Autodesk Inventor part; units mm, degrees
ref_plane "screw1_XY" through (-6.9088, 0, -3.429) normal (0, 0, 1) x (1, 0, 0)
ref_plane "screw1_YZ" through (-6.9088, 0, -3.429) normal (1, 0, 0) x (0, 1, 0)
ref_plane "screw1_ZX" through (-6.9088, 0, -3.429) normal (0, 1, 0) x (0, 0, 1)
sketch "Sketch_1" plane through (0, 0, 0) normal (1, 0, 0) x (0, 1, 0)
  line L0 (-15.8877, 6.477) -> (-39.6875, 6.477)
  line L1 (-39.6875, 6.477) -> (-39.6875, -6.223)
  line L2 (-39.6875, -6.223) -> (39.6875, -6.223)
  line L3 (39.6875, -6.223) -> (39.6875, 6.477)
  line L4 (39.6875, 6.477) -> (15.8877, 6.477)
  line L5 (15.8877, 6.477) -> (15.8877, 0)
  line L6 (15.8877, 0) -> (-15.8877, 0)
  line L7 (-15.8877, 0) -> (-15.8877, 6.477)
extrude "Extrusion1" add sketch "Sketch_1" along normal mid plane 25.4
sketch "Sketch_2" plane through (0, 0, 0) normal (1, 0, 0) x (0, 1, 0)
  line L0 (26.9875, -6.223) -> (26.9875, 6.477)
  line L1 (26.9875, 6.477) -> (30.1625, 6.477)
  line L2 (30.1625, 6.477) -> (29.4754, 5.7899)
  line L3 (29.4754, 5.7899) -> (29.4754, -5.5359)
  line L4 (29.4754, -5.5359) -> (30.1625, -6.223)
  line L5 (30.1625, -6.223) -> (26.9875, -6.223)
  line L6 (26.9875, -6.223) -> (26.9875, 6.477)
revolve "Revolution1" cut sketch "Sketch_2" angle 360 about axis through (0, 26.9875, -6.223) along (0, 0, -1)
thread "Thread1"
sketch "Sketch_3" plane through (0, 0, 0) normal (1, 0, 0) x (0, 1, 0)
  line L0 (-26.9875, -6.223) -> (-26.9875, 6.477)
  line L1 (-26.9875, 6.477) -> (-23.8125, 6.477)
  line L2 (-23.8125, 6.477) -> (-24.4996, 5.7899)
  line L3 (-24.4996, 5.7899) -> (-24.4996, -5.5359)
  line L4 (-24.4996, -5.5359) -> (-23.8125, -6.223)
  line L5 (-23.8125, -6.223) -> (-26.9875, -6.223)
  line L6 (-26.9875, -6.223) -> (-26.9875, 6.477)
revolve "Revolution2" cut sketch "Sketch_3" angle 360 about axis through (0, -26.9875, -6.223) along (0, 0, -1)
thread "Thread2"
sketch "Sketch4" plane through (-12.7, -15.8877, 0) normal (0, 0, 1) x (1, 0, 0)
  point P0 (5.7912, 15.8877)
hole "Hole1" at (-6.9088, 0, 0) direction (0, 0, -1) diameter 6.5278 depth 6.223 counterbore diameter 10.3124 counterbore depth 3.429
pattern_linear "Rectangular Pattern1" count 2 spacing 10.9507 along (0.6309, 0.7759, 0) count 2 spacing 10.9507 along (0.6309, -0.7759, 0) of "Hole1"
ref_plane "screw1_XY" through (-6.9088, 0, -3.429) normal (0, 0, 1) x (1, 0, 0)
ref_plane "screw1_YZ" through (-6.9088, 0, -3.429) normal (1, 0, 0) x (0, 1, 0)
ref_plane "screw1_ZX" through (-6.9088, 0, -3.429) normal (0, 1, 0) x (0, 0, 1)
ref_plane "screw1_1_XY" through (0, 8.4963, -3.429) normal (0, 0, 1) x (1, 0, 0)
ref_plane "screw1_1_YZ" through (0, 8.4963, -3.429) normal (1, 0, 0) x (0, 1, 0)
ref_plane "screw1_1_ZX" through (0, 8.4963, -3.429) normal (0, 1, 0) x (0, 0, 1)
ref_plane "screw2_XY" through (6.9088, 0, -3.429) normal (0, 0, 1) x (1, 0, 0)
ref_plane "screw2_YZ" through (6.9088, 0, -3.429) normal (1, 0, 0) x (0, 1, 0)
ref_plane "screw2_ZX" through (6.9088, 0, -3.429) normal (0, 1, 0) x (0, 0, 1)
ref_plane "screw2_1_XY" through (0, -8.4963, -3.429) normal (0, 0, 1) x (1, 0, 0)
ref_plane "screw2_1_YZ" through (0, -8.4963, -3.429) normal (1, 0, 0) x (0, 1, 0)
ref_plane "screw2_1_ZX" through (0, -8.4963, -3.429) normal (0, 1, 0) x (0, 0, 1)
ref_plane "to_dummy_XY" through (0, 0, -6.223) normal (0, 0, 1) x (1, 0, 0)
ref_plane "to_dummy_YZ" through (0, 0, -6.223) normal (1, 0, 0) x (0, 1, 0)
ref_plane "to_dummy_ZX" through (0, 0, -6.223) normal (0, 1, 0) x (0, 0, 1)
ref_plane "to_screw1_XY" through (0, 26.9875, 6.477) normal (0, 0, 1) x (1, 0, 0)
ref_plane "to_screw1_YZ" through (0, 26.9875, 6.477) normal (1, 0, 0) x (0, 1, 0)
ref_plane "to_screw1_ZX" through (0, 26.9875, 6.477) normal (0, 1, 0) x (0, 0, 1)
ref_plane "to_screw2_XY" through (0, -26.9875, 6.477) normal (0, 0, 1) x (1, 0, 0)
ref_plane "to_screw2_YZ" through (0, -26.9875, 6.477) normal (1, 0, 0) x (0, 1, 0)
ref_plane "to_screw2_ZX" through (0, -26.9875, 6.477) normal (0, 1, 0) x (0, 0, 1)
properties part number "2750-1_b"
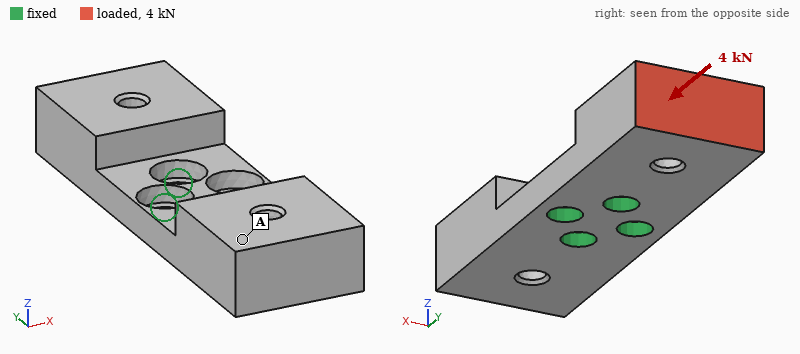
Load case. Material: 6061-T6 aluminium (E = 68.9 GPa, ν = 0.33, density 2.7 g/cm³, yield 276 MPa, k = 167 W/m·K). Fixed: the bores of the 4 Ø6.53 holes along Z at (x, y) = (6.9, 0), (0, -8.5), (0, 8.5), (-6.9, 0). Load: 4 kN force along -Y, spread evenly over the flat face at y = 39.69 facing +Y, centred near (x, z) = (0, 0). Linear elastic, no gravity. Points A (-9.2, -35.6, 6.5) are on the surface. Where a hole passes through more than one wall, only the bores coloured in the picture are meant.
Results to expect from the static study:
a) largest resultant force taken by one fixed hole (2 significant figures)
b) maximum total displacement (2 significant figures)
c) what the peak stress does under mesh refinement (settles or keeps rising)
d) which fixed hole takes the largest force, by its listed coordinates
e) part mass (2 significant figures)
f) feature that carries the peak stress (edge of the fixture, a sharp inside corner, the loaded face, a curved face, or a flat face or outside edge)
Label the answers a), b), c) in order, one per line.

a) 1.8 kN
b) 0.20 mm
c) keeps rising
d) (0, 8.5)
e) 50 g
f) edge of the fixture
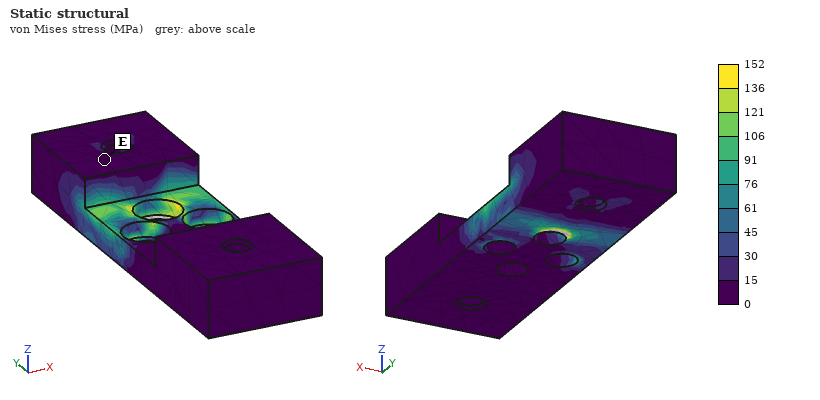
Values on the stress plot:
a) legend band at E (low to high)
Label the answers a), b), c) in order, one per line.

a) 0 to 15 MPa
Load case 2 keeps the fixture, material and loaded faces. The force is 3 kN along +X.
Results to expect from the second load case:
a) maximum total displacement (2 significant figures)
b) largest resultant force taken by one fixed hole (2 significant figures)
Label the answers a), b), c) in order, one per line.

a) 0.13 mm
b) 4.2 kN
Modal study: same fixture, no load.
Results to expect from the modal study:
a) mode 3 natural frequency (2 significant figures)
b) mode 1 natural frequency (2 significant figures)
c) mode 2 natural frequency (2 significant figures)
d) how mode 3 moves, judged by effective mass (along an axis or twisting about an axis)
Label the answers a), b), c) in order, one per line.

a) 7200 Hz
b) 3000 Hz
c) 3000 Hz
d) twisting about Z
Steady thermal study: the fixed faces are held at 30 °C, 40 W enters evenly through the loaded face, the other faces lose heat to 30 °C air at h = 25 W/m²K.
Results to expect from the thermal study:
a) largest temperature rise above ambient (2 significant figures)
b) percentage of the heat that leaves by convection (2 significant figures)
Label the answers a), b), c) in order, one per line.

a) 37 K
b) 4.0 %
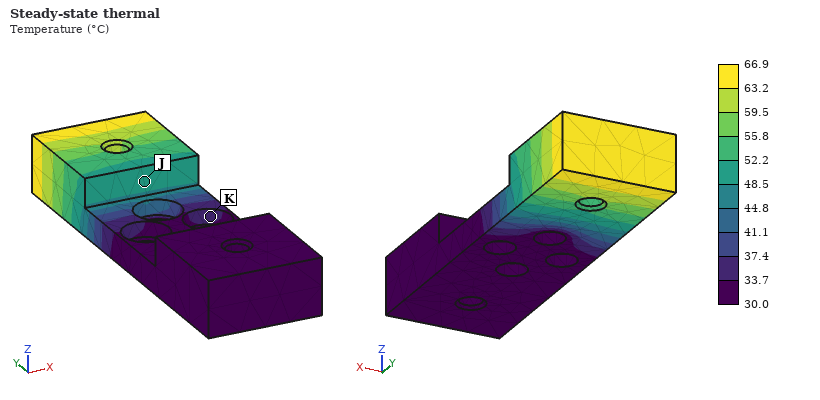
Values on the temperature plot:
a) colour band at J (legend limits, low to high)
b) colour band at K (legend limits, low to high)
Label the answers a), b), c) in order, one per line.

a) 48.5 to 52.2 °C
b) 33.7 to 37.4 °C
